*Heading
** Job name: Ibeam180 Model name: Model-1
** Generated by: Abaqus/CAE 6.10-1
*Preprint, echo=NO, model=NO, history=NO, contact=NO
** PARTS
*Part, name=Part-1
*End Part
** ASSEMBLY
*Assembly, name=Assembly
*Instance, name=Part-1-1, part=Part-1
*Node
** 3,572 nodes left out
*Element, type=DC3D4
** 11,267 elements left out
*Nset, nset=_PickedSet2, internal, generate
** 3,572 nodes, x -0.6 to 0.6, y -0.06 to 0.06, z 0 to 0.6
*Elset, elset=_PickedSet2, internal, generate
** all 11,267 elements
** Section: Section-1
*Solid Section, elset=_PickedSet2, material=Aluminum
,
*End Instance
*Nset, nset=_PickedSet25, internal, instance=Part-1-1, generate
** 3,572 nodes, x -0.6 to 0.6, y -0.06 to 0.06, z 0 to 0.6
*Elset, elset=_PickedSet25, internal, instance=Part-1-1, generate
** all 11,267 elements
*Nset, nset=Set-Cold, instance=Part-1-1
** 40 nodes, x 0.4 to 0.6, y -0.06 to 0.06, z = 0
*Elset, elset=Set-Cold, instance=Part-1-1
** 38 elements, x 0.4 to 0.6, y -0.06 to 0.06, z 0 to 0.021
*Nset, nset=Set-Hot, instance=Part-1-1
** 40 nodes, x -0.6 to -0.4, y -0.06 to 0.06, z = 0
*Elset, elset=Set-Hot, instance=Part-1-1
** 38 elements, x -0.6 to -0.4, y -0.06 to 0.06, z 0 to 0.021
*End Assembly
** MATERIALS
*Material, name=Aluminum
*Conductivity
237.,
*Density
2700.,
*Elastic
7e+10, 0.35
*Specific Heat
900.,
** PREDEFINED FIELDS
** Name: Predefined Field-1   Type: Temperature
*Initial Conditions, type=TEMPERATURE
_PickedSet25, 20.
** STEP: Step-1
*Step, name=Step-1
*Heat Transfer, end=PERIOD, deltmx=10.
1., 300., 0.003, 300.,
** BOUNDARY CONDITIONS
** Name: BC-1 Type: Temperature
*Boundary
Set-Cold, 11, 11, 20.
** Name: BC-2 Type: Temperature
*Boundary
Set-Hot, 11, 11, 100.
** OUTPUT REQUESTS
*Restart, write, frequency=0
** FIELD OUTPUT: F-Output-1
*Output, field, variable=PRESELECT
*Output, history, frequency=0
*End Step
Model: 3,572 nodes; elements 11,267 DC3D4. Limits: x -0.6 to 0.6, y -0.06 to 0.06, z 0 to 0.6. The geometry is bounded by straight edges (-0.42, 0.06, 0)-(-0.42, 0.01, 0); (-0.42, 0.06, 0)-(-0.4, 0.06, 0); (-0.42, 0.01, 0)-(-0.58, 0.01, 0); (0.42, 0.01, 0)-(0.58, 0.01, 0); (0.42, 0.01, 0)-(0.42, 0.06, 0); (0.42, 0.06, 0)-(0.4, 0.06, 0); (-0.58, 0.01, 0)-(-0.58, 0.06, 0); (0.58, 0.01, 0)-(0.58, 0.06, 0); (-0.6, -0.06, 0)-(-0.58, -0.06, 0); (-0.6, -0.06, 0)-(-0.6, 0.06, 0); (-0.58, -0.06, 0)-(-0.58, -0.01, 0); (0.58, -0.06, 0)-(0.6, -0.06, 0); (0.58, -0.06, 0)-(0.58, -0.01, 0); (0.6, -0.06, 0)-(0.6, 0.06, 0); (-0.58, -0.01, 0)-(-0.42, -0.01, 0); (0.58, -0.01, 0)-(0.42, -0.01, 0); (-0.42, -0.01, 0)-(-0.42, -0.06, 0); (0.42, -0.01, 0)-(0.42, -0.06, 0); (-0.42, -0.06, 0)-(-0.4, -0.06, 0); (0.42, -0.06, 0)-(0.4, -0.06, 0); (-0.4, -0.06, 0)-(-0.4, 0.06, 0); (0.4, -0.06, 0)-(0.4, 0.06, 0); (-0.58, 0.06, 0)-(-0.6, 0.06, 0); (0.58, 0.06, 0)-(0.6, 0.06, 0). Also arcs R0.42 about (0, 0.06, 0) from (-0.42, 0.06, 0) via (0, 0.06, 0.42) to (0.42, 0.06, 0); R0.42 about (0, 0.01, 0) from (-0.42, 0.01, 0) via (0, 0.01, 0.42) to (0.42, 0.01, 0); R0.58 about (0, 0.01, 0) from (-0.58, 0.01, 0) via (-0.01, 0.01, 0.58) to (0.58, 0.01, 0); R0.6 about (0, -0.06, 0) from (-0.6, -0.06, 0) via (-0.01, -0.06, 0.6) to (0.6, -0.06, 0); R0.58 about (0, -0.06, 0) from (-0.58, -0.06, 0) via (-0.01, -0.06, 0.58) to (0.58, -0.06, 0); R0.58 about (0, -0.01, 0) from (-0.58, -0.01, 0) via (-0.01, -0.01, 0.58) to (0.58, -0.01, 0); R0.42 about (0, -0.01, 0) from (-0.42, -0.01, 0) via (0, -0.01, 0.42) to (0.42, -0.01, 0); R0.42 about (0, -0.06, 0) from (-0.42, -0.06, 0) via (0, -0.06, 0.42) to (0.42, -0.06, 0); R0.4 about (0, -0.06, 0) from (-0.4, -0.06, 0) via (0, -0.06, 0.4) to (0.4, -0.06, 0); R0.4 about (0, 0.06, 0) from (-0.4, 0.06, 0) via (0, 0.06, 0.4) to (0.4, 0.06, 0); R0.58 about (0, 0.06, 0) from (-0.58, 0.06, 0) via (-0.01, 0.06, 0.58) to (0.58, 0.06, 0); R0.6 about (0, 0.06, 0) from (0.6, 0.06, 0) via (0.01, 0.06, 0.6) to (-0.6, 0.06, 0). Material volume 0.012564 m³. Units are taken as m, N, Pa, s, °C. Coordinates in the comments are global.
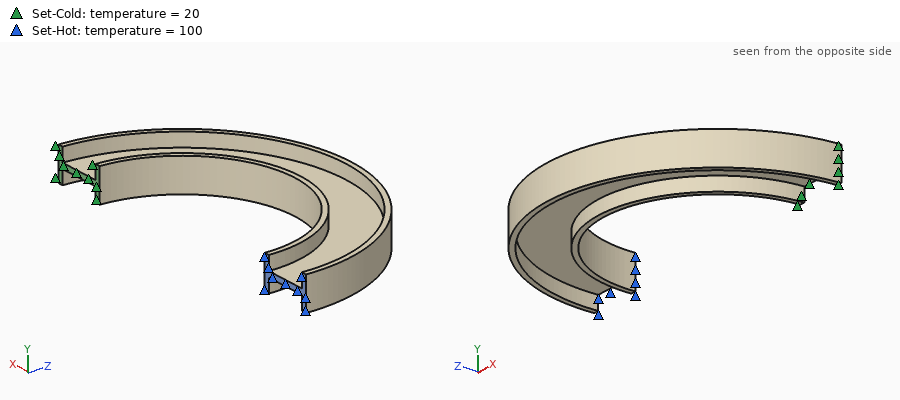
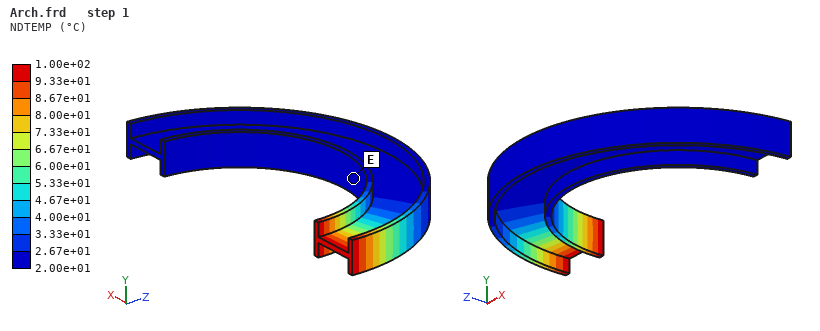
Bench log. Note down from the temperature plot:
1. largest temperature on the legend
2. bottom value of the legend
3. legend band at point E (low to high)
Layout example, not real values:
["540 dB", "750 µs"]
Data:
["1.00e+02 °C", "2.00e+01 °C", "2.00e+01 to 2.67e+01 °C"]
